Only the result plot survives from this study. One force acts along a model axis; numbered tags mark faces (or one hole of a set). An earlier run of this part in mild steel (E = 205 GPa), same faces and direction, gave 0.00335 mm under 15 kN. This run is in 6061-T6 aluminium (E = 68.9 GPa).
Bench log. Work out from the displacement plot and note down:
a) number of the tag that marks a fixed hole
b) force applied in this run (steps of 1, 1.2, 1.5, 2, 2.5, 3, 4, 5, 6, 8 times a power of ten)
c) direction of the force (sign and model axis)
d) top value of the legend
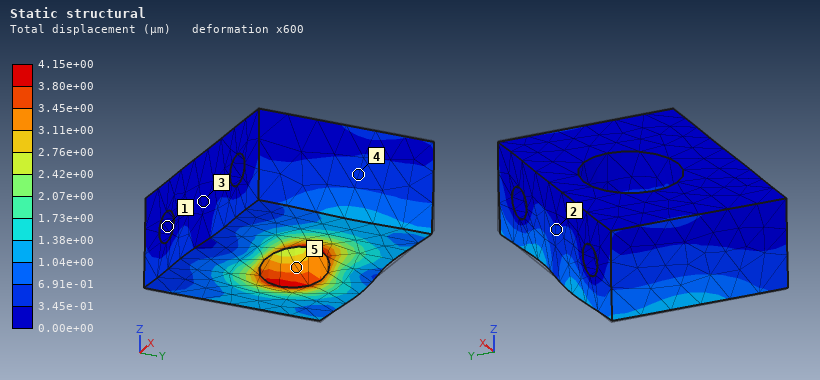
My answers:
1
6 kN
-X
4.15e+00 µm
